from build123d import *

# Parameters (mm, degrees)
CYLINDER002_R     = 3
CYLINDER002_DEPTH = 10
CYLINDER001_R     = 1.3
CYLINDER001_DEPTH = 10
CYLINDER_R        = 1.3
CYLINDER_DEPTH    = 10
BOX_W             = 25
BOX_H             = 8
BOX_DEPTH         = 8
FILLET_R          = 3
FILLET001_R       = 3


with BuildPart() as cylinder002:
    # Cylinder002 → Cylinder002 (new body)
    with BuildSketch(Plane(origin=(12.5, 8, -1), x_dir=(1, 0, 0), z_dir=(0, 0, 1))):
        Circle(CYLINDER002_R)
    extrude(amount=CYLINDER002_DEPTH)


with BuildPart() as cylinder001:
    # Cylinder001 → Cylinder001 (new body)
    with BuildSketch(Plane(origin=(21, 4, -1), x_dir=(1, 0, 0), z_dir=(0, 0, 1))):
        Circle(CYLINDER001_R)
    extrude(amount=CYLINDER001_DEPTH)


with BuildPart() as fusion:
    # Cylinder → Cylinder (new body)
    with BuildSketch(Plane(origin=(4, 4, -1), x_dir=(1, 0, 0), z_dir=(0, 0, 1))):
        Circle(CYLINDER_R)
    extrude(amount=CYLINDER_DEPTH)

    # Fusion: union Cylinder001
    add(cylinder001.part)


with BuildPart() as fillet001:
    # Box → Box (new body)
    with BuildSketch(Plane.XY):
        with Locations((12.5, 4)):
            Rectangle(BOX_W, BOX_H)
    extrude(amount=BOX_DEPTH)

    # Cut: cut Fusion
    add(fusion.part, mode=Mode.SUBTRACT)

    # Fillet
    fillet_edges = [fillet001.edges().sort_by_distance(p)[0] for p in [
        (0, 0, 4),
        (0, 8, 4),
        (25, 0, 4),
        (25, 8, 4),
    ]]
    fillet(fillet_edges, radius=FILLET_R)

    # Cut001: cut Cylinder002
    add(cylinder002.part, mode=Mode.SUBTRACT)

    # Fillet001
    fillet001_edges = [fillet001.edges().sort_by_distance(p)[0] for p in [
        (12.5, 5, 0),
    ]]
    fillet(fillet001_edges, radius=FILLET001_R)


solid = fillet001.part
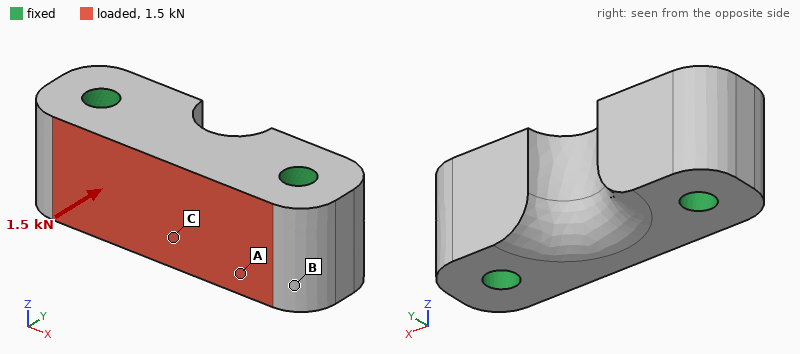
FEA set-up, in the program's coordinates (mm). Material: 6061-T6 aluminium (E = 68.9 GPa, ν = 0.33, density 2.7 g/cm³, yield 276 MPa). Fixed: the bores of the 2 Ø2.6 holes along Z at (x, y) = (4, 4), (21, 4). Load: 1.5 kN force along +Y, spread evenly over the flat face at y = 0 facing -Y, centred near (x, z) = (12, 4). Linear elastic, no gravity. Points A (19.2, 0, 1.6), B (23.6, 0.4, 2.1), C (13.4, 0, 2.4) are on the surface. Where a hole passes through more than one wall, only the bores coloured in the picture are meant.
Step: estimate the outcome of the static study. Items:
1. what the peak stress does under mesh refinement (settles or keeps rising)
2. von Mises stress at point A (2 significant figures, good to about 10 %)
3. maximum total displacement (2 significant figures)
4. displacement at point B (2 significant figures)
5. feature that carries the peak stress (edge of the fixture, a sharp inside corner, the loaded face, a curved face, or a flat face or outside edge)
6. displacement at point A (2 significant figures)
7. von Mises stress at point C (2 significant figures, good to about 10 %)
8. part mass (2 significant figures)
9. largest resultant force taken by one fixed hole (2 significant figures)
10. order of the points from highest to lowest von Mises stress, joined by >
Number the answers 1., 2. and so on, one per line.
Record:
1. keeps rising
2. 13 MPa
3. 4.5 µm
4. 0.87 µm
5. edge of the fixture
6. 1.9 µm
7. 25 MPa
8. 3.6 g
9. 810 N
10. C > A > B
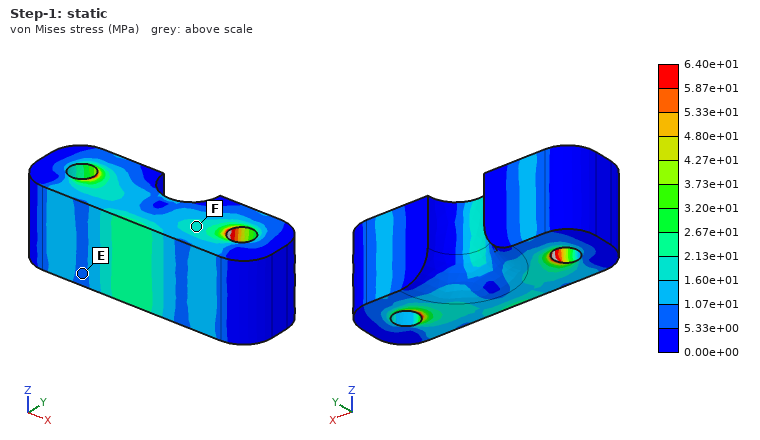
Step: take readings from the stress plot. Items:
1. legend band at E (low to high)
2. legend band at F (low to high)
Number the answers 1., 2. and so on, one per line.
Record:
1. 5.33e+00 to 1.07e+01 MPa
2. 1.60e+01 to 2.13e+01 MPa
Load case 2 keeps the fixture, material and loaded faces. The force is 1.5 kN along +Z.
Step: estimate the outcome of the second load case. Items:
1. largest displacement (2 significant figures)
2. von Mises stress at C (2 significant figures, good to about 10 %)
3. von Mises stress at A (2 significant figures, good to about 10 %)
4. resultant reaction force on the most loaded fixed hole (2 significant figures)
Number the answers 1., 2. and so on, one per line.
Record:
1. 8.2 µm
2. 21 MPa
3. 35 MPa
4. 750 N
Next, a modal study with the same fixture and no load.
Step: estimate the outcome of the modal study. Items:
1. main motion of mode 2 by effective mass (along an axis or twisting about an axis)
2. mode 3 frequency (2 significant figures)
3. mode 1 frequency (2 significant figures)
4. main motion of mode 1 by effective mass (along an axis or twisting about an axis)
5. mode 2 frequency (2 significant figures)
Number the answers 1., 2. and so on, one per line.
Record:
1. along Z
2. 110 kHz
3. 66 kHz
4. along Y
5. 79 kHz
